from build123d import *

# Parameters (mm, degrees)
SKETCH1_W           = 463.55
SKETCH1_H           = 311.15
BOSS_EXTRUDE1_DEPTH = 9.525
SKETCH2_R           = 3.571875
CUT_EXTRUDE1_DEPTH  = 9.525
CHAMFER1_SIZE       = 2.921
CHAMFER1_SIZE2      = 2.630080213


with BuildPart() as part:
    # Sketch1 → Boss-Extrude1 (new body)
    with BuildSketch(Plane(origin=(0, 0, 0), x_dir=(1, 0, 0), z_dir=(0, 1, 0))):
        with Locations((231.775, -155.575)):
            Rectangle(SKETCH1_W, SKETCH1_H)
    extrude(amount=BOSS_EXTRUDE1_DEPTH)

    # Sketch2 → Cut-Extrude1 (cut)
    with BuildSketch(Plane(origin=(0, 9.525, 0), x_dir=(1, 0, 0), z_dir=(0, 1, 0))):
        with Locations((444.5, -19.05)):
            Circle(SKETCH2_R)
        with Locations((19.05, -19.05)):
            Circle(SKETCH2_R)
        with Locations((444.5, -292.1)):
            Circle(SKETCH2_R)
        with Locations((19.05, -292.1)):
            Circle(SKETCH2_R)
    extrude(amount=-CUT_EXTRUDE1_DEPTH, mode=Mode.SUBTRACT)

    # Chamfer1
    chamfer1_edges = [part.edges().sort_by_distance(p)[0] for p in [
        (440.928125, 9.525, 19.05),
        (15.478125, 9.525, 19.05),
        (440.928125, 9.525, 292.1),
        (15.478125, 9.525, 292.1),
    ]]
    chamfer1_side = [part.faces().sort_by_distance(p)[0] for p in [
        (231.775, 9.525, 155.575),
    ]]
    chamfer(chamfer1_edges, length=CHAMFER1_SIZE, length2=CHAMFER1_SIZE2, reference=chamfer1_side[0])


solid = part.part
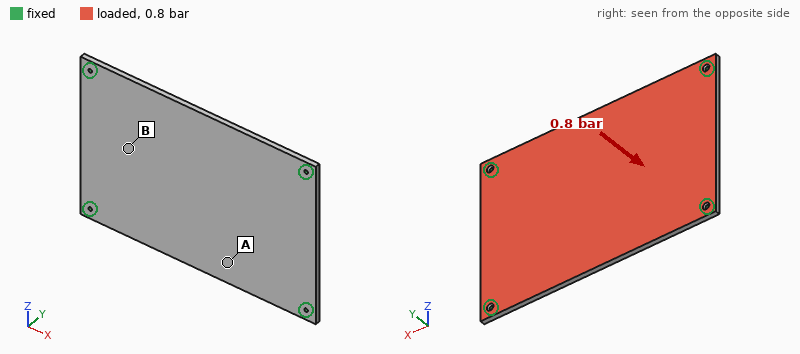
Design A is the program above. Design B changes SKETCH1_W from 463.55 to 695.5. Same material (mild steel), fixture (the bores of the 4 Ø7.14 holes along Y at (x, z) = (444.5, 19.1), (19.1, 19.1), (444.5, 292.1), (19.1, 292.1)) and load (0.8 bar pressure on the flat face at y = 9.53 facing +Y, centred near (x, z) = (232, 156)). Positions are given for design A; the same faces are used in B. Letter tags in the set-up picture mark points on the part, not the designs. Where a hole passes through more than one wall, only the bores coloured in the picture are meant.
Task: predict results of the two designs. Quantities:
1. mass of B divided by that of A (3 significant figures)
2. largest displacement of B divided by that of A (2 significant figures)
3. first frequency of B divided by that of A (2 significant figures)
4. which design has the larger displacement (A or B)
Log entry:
1.50
0.78
0.96
A
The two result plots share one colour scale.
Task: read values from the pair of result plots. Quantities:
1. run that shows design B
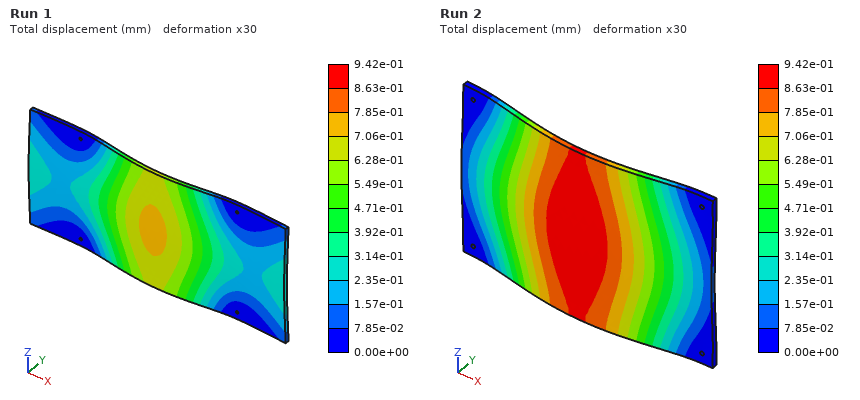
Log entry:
Run 1
